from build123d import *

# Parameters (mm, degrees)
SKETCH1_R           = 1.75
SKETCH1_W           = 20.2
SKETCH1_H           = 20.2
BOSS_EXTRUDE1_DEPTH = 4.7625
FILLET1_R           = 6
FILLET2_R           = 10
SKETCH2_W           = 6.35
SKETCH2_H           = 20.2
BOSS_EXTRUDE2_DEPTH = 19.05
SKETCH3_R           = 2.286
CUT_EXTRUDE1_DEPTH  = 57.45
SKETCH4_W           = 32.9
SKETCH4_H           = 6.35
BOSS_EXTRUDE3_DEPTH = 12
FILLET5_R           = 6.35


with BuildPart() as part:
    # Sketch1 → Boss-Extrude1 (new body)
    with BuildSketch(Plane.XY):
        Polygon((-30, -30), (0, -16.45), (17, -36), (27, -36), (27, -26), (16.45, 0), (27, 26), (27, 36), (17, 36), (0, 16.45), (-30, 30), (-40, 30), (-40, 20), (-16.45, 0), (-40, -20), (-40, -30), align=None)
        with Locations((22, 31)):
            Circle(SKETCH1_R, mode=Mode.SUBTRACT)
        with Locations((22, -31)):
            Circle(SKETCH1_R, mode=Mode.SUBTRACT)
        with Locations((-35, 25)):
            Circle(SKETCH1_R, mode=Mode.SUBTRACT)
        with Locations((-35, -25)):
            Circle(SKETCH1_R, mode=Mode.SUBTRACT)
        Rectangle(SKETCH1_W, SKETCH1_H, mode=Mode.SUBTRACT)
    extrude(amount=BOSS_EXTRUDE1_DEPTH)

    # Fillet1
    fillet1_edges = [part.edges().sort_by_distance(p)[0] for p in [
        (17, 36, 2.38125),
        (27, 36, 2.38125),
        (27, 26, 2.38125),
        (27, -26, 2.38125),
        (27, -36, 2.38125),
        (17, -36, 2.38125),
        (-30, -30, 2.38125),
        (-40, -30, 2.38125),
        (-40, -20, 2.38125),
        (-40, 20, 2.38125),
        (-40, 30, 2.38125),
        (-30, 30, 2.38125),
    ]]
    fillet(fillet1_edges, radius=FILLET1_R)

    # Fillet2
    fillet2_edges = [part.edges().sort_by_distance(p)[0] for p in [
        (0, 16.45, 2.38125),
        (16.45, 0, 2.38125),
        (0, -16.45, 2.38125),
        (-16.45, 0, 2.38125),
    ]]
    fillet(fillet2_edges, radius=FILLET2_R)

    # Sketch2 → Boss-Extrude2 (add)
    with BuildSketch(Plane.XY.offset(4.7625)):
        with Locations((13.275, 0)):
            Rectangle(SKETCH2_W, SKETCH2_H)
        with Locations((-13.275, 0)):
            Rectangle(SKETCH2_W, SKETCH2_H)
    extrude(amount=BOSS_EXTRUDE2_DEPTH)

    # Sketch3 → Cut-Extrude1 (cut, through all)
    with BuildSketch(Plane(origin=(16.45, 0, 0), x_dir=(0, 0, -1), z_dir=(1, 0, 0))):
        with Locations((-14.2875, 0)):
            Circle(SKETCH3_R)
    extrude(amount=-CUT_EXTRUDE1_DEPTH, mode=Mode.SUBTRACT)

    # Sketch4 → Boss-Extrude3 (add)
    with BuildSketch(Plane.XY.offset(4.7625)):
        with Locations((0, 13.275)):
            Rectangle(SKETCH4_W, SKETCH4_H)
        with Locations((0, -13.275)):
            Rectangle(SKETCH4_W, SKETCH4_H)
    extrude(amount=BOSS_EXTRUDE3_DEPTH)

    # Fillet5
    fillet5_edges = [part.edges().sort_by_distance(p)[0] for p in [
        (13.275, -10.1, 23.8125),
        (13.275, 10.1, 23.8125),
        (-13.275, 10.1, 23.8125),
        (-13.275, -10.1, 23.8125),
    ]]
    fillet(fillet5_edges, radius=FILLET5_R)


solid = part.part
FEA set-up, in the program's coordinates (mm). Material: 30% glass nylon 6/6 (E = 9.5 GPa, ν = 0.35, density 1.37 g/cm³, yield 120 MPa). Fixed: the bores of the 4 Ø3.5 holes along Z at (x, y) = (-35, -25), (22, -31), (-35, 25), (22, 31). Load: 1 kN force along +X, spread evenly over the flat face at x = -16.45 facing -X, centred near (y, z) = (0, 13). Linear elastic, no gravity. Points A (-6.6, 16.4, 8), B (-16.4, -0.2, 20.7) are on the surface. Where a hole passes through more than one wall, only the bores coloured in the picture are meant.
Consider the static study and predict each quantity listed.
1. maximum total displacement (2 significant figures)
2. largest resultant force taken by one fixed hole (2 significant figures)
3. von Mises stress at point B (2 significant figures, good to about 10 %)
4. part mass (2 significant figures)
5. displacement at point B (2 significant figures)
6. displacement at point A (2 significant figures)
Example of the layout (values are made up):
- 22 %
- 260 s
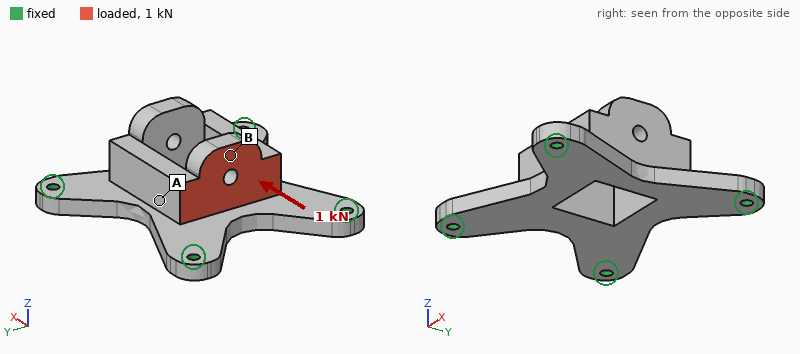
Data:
- 0.19 mm
- 360 N
- 8.6 MPa
- 29 g
- 0.16 mm
- 0.042 mm
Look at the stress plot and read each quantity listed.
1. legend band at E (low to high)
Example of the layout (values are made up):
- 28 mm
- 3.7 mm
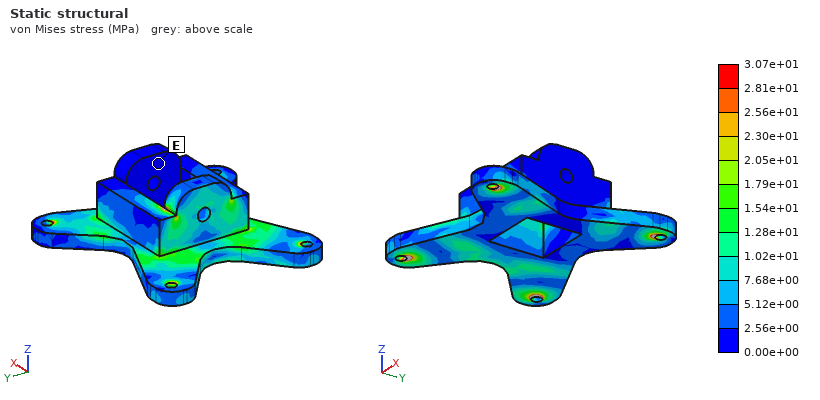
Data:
- 0.00e+00 to 2.56e+00 MPa
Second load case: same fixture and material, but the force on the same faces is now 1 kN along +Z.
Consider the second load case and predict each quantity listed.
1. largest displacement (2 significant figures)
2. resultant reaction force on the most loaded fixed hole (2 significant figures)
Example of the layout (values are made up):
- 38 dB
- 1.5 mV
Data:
- 0.37 mm
- 390 N
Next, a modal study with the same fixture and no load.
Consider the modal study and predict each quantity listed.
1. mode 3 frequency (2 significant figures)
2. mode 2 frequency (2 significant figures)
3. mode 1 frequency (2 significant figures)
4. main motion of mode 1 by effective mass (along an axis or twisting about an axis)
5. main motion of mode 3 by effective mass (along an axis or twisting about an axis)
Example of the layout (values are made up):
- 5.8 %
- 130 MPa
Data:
- 3800 Hz
- 3600 Hz
- 2400 Hz
- along Z
- along Y
